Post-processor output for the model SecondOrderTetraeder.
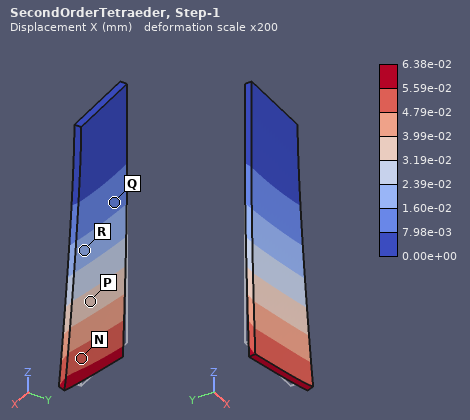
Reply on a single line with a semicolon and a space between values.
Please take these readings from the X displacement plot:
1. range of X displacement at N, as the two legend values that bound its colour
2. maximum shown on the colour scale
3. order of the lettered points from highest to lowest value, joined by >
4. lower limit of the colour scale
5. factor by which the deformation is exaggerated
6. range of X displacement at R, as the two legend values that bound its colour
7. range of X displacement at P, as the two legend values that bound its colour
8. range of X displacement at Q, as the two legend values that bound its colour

4.79e-02 to 5.59e-02 mm; 6.38e-02 mm; N > P > R > Q; 0.00e+00 mm; 200; 1.60e-02 to 2.39e-02 mm; 3.19e-02 to 3.99e-02 mm; 7.98e-03 to 1.60e-02 mm
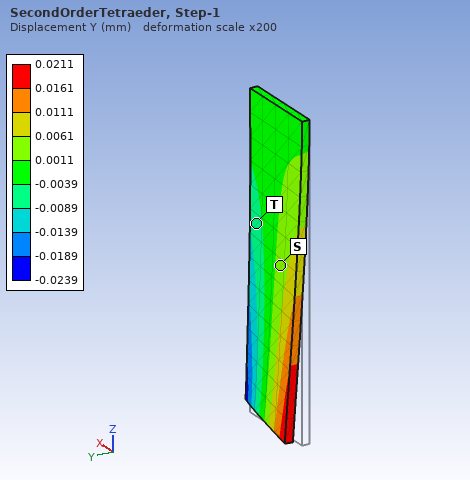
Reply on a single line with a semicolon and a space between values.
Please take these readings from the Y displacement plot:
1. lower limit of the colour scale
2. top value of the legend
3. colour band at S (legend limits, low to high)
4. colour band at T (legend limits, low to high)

-0.0239 mm; 0.0211 mm; 0.0011 to 0.0061 mm; -0.0089 to -0.0039 mm
